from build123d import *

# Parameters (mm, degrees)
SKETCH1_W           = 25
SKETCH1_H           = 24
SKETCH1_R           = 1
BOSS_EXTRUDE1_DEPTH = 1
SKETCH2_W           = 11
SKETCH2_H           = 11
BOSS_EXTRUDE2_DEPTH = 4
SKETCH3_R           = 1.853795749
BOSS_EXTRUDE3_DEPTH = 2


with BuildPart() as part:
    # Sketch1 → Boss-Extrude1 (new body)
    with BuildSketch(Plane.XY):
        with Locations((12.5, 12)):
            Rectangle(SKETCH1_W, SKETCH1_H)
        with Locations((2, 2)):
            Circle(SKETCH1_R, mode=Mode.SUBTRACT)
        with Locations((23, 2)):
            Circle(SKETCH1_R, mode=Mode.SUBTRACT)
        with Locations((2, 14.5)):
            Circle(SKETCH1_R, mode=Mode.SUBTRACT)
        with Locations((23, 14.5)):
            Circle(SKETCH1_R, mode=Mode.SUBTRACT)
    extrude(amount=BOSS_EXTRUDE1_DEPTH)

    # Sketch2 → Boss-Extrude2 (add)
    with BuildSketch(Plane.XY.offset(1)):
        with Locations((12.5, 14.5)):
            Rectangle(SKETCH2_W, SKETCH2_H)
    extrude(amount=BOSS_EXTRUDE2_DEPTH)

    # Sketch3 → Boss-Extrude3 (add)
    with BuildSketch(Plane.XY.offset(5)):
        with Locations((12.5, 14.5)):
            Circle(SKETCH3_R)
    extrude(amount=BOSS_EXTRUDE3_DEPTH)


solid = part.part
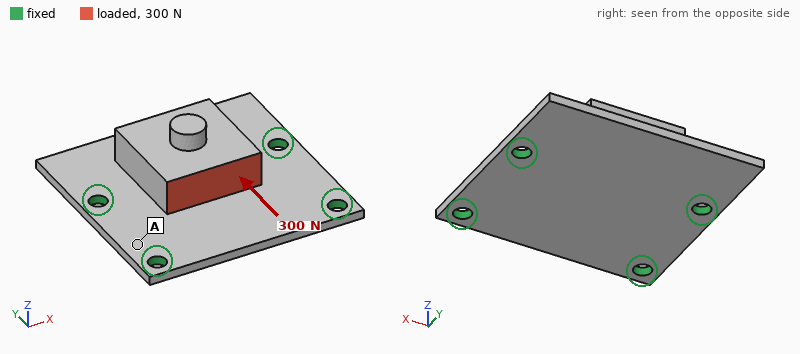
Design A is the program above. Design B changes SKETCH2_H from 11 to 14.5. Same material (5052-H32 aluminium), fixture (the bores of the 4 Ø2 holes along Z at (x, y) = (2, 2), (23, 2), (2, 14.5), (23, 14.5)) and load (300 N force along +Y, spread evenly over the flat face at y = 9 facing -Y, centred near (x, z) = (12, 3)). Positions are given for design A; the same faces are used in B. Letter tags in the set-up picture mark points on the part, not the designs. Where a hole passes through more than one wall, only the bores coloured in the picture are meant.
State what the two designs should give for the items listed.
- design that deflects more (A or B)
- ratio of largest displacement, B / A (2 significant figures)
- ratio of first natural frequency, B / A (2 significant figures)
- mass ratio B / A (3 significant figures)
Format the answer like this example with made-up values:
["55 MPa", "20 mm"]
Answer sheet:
["A", "0.73", "0.95", "1.14"]
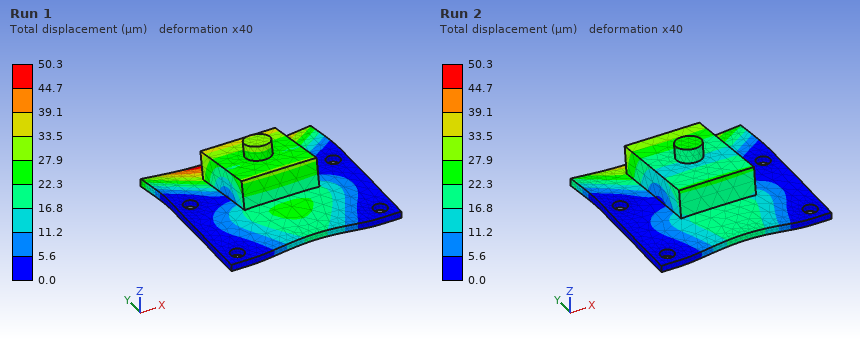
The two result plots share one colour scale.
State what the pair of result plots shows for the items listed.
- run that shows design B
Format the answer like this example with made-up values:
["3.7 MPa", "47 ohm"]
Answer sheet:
["Run 2"]
